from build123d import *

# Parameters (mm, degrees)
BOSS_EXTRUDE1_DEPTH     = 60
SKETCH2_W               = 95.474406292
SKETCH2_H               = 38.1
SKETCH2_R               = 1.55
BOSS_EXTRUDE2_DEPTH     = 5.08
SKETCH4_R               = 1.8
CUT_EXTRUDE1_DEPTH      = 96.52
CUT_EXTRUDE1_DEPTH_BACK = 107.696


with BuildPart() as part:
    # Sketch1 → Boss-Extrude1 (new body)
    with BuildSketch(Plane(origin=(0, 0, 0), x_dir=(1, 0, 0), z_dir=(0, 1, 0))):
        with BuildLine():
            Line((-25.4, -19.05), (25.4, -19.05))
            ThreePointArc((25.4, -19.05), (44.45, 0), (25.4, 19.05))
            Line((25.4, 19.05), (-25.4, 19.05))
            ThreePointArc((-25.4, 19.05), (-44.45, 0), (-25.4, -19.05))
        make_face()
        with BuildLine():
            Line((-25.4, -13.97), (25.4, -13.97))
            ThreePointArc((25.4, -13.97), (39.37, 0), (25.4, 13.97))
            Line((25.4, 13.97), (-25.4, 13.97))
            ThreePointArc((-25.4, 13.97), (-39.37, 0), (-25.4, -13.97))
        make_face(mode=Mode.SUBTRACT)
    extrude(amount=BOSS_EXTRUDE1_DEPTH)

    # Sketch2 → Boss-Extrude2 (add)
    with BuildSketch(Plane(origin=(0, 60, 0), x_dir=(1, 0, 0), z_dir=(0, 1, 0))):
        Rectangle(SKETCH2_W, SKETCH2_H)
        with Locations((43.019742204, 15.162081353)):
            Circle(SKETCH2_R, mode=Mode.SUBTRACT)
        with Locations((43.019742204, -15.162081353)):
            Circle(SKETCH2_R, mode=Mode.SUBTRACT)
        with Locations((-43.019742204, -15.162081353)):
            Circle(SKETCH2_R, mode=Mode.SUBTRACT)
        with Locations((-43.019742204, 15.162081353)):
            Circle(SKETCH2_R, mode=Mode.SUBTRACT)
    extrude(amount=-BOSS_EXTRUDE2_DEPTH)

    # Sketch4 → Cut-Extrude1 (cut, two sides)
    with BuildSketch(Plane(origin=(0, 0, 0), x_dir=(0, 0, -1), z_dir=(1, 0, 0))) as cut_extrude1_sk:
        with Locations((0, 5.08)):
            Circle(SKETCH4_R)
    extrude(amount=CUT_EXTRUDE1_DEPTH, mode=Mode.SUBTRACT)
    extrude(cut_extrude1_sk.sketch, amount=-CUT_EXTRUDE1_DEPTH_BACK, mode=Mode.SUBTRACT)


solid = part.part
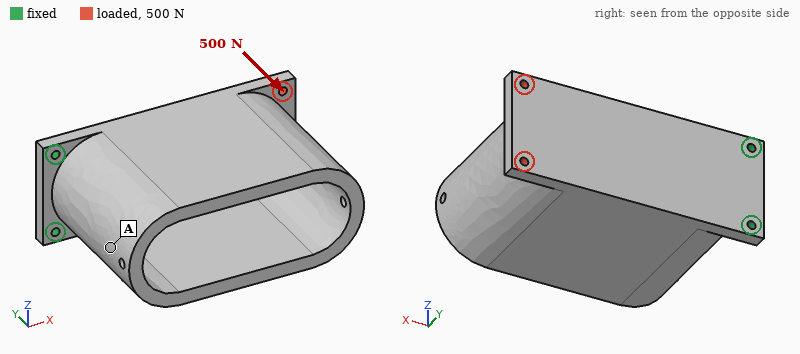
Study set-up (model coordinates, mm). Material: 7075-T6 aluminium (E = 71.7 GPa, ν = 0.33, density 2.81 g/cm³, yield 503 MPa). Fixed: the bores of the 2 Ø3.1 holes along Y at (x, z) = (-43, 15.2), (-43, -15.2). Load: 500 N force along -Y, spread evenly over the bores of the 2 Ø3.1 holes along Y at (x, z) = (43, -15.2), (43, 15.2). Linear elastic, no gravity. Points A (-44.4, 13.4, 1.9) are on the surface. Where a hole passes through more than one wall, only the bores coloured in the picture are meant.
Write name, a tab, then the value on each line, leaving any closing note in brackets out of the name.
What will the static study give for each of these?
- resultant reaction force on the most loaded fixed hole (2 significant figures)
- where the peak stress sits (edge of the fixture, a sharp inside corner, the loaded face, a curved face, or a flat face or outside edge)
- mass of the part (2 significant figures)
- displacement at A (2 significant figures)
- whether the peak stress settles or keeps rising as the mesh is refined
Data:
resultant reaction force on the most loaded fixed hole	330 N
where the peak stress sits	edge of the fixture
mass of the part	210 g
displacement at A	0.51 mm
whether the peak stress settles or keeps rising as the mesh is refined	keeps rising
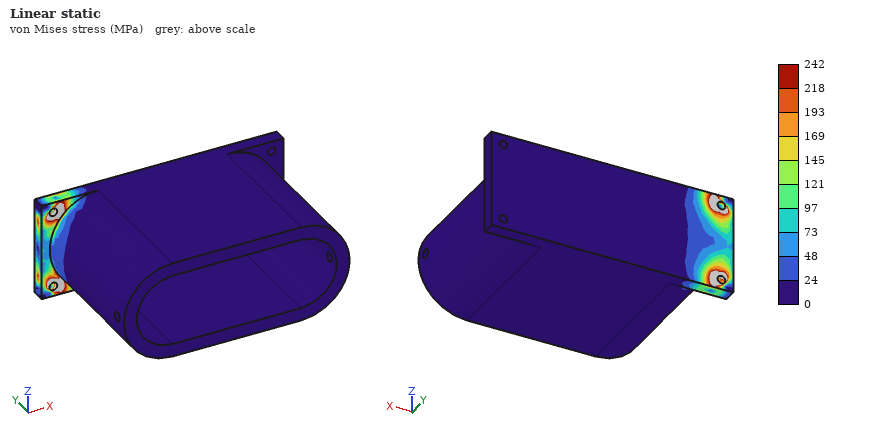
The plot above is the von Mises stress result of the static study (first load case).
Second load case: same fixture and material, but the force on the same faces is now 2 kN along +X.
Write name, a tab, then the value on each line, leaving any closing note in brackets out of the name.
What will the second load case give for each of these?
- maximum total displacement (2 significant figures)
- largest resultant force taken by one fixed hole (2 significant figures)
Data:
maximum total displacement	22 µm
largest resultant force taken by one fixed hole	1.0 kN
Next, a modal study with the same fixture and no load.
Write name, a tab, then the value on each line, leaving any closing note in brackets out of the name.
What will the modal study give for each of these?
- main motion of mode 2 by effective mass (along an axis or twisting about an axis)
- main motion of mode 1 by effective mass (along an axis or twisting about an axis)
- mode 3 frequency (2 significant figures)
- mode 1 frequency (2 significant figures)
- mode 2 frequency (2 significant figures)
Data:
main motion of mode 2 by effective mass	along Z
main motion of mode 1 by effective mass	along Y
mode 3 frequency	2600 Hz
mode 1 frequency	360 Hz
mode 2 frequency	1300 Hz
